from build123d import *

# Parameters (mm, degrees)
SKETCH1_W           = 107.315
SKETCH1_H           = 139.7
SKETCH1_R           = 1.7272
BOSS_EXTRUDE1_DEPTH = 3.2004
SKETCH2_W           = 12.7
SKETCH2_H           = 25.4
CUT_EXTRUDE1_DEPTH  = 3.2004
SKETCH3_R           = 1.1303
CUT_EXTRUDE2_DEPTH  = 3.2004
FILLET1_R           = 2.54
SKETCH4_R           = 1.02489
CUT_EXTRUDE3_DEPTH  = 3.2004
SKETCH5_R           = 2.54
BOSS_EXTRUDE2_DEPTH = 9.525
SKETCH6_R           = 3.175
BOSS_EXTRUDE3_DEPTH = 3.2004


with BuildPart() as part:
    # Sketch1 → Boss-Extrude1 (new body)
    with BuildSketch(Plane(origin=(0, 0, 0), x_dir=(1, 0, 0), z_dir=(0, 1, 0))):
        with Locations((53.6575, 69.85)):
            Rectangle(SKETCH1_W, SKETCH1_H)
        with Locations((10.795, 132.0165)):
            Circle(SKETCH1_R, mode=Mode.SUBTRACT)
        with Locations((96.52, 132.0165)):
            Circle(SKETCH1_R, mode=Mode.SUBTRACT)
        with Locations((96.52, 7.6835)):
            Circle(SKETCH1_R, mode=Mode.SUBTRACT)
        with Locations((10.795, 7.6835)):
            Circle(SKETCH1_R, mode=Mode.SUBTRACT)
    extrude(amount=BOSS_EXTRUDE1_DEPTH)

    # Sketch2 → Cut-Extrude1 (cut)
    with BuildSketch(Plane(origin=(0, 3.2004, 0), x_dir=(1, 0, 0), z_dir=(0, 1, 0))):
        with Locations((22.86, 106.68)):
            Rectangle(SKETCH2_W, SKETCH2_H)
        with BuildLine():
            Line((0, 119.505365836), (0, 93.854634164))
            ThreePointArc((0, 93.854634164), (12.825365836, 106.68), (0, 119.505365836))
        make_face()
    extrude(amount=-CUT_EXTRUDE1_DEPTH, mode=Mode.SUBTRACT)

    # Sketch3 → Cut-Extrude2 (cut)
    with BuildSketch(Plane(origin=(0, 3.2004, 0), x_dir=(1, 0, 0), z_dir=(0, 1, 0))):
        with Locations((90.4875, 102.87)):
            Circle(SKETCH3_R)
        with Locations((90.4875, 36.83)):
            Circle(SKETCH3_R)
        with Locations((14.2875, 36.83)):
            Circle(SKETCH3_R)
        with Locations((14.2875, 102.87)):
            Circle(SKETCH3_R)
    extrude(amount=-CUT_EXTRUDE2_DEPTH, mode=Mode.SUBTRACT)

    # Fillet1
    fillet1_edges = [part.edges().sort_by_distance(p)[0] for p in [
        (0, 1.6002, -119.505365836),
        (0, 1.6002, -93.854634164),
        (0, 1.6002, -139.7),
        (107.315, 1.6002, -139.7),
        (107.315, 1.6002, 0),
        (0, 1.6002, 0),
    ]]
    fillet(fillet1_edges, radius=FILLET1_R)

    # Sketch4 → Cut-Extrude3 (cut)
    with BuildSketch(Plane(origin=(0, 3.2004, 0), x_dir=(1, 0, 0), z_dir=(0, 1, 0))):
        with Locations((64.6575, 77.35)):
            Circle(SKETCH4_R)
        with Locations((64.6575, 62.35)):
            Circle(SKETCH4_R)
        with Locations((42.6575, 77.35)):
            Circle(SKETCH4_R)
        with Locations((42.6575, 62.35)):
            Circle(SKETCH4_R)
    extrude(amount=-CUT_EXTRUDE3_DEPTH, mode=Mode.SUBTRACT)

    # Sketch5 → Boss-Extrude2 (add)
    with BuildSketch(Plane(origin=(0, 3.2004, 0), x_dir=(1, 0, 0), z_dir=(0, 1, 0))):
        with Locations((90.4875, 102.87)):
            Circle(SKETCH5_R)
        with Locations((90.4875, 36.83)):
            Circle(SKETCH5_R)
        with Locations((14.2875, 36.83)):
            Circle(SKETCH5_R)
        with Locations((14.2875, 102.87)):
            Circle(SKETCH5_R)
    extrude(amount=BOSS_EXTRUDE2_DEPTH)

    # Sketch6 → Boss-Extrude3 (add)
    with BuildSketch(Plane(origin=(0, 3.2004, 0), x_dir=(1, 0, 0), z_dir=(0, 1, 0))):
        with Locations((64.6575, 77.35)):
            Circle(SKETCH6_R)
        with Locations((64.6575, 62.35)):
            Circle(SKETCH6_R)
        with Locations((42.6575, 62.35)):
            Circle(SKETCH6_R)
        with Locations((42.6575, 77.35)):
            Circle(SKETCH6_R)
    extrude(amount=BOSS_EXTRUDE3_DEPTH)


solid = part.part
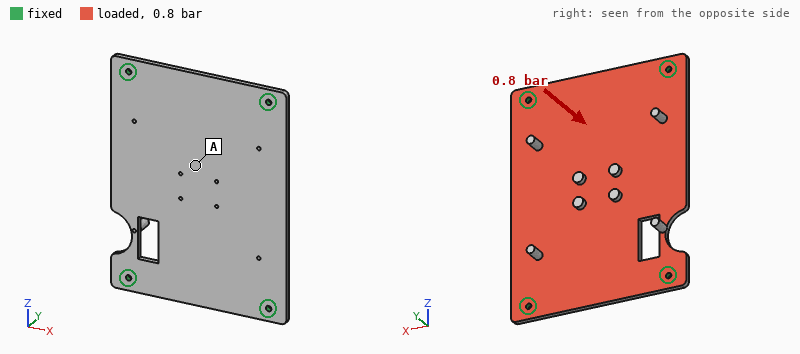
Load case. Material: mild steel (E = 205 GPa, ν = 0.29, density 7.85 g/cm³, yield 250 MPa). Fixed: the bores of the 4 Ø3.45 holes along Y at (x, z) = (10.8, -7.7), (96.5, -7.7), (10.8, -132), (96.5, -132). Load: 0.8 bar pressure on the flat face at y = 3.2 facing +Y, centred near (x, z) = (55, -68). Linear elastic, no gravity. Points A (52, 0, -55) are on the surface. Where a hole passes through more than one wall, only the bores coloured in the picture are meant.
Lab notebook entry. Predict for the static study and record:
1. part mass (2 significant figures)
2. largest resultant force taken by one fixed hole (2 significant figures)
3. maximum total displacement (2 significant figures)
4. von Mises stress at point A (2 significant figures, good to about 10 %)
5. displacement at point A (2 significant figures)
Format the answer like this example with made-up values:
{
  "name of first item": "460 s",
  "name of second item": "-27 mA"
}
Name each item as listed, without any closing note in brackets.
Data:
{
  "part mass": "370 g",
  "largest resultant force taken by one fixed hole": "300 N",
  "maximum total displacement": "0.15 mm",
  "von Mises stress at point A": "28 MPa",
  "displacement at point A": "0.14 mm"
}
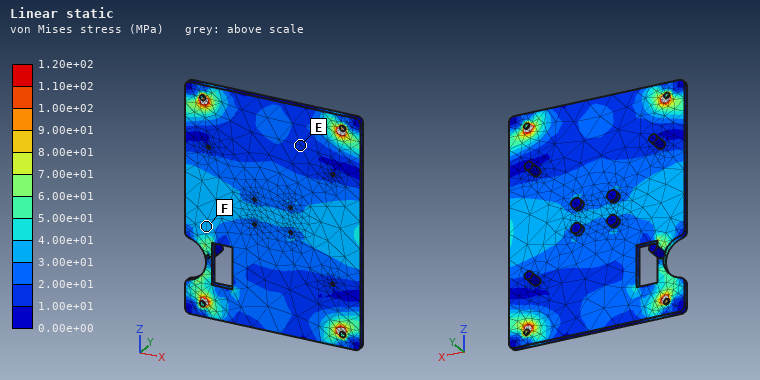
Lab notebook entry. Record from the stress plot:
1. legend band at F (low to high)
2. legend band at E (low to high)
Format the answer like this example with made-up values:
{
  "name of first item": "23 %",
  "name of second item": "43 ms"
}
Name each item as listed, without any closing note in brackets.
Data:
{
  "legend band at F": "3.00e+01 to 4.00e+01 MPa",
  "legend band at E": "1.00e+01 to 2.00e+01 MPa"
}
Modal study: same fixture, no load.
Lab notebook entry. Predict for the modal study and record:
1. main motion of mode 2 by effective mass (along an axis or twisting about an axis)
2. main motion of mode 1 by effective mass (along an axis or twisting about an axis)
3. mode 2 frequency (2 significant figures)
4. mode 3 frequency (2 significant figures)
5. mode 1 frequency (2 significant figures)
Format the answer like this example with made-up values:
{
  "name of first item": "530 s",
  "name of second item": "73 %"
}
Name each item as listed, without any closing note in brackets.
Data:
{
  "main motion of mode 2 by effective mass": "twisting about Z",
  "main motion of mode 1 by effective mass": "along Y",
  "mode 2 frequency": "1300 Hz",
  "mode 3 frequency": "2000 Hz",
  "mode 1 frequency": "830 Hz"
}
